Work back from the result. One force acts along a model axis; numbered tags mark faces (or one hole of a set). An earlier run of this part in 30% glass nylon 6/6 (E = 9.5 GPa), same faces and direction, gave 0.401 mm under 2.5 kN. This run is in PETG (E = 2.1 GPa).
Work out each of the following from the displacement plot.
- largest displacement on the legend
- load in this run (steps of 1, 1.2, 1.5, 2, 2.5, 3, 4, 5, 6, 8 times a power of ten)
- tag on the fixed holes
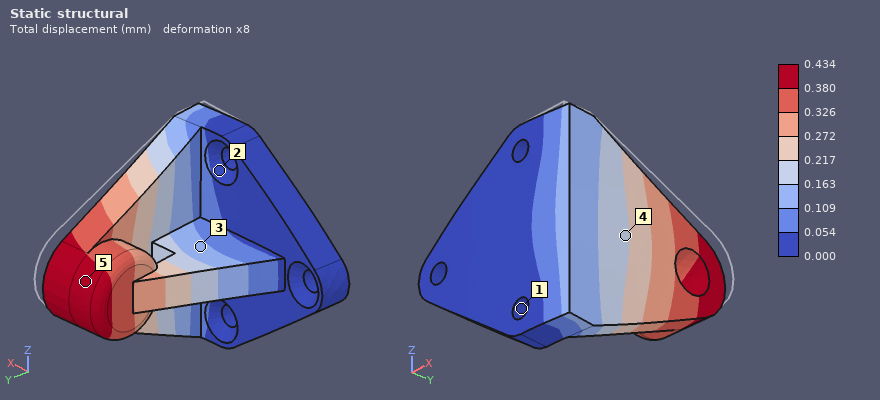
0.434 mm
600 N
1
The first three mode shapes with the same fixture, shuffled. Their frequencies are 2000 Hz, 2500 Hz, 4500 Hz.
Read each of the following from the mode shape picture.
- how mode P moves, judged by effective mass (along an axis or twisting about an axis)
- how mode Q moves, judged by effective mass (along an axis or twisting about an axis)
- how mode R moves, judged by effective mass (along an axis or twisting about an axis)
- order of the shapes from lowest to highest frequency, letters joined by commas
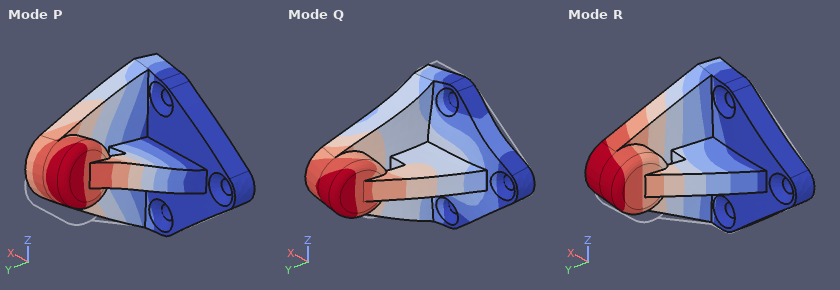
along Z
along Y
along X
R, P, Q
